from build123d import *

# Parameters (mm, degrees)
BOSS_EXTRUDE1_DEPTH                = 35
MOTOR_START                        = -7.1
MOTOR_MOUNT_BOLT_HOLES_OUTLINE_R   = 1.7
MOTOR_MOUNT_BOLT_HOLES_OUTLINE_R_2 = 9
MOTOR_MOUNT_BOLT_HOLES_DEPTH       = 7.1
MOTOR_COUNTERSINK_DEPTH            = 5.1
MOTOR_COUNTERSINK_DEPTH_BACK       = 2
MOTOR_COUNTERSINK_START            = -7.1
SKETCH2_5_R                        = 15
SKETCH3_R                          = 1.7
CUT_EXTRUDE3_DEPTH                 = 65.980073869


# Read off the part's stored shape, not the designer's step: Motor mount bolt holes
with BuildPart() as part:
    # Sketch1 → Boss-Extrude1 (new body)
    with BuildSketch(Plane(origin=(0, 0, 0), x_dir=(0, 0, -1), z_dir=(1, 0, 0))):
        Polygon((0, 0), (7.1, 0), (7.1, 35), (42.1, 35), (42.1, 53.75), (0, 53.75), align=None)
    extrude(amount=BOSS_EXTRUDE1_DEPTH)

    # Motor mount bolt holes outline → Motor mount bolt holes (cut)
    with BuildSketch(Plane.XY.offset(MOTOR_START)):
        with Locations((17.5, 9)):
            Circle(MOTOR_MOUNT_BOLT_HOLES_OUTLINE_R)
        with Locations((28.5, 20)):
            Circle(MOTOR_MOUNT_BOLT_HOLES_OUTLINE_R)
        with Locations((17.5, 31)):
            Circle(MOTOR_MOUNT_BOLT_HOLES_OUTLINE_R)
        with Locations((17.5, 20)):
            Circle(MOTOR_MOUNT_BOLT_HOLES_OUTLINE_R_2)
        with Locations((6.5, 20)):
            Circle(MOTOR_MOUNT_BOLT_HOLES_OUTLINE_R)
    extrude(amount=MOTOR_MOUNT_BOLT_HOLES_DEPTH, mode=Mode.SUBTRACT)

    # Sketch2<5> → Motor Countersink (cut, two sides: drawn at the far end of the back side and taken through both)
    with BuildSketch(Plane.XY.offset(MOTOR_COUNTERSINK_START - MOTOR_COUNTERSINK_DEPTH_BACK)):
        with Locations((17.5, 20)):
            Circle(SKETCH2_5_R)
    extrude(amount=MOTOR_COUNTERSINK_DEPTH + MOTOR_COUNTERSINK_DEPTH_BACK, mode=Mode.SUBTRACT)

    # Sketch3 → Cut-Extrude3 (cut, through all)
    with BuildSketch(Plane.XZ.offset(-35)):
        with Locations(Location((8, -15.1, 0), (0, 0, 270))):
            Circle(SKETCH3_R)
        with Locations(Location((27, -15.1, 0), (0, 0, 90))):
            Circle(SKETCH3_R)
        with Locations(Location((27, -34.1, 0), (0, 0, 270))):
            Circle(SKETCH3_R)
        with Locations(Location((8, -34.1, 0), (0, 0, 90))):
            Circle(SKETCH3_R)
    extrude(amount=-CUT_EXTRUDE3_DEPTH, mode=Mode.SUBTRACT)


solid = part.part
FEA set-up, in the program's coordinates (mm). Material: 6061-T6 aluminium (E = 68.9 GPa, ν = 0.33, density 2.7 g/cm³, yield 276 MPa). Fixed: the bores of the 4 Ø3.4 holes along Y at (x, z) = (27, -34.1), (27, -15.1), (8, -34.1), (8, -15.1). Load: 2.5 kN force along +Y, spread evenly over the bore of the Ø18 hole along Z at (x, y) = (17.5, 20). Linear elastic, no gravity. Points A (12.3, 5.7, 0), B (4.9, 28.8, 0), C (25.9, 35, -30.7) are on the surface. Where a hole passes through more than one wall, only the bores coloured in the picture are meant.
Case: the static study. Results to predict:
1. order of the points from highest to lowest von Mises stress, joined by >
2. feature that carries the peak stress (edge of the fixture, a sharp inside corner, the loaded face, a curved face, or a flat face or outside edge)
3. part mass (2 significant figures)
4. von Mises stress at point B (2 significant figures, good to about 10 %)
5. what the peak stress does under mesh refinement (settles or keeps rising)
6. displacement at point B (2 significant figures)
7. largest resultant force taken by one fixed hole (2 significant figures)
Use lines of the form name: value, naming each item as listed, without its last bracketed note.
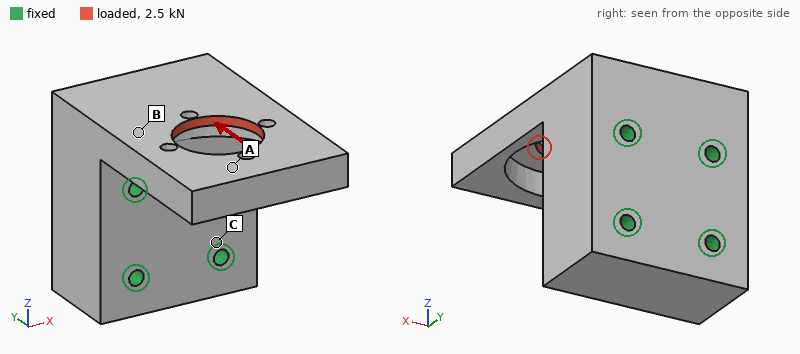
order of the points from highest to lowest von Mises stress, joined by >: B > A > C
feature that carries the peak stress: a sharp inside corner
part mass: 85 g
von Mises stress at point B: 42 MPa
what the peak stress does under mesh refinement: keeps rising
displacement at point B: 16 µm
largest resultant force taken by one fixed hole: 1.4 kN
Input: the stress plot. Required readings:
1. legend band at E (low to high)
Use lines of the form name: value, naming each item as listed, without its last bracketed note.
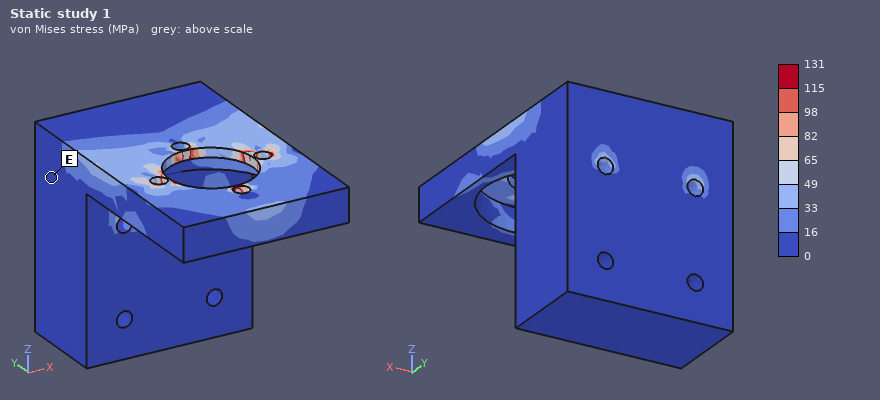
legend band at E: 0 to 16 MPa
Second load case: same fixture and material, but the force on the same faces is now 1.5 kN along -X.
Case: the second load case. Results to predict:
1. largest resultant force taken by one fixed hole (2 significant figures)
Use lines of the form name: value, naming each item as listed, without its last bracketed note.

largest resultant force taken by one fixed hole: 1.5 kN
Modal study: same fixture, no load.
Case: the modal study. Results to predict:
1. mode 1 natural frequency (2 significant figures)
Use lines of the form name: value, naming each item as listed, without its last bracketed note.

mode 1 natural frequency: 2700 Hz
